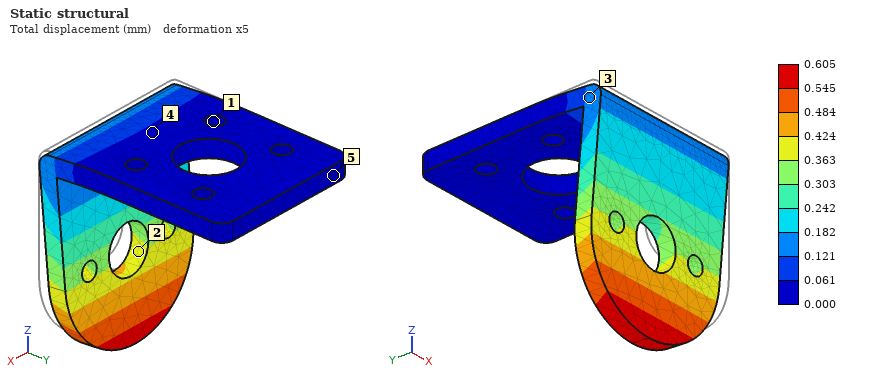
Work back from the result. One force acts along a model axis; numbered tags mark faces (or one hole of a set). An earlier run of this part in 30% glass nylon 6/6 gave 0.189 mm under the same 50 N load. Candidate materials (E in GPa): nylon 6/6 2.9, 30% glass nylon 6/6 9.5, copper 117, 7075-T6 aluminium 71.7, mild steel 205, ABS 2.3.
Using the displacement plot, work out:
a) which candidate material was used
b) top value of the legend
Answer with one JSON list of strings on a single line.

["nylon 6/6", "0.605 mm"]
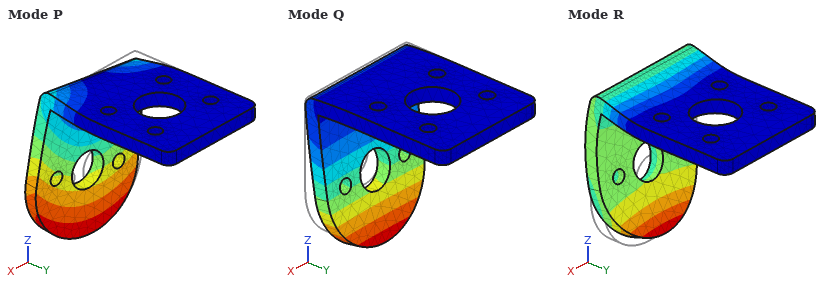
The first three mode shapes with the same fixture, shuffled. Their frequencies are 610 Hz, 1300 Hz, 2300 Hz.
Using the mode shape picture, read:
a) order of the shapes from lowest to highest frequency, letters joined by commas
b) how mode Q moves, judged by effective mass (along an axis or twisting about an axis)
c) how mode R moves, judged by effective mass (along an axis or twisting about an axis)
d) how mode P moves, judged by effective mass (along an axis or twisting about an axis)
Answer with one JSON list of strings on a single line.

["Q, P, R", "along Y", "along Z", "along X"]
